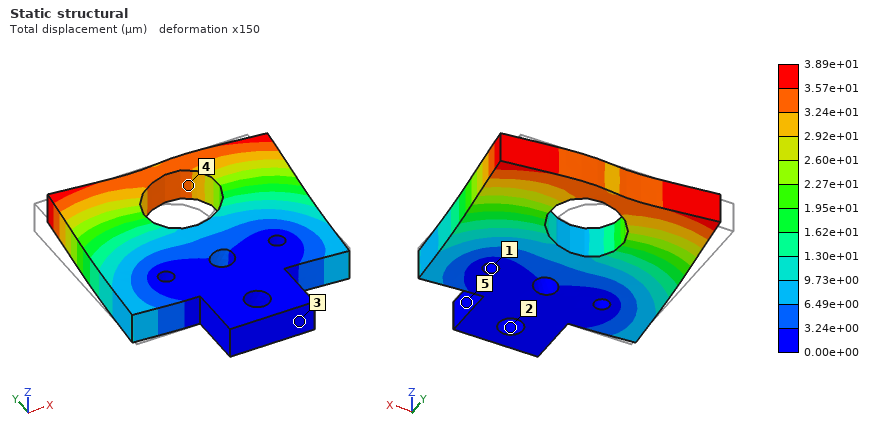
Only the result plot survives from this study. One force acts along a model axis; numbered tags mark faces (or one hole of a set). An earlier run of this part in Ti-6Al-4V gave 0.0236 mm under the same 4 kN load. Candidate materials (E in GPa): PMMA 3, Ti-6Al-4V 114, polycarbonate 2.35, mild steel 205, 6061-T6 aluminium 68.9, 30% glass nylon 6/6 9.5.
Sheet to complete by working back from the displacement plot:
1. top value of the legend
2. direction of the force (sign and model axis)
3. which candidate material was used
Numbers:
3.89e+01 µm
+X
6061-T6 aluminium
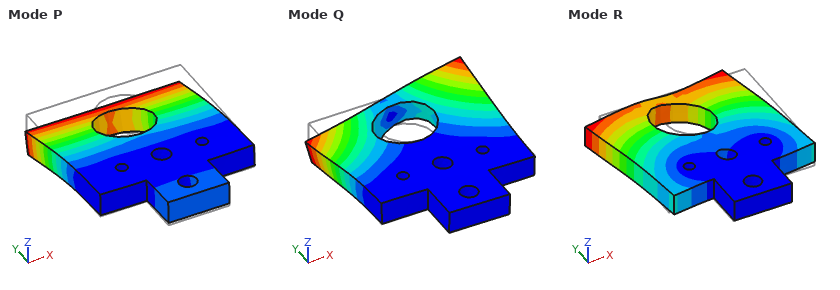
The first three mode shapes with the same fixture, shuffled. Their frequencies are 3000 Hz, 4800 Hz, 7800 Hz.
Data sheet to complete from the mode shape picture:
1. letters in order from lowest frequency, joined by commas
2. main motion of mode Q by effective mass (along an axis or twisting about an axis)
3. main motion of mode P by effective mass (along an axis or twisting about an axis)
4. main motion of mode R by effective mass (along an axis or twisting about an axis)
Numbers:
P, Q, R
twisting about Y
along Z
along X
